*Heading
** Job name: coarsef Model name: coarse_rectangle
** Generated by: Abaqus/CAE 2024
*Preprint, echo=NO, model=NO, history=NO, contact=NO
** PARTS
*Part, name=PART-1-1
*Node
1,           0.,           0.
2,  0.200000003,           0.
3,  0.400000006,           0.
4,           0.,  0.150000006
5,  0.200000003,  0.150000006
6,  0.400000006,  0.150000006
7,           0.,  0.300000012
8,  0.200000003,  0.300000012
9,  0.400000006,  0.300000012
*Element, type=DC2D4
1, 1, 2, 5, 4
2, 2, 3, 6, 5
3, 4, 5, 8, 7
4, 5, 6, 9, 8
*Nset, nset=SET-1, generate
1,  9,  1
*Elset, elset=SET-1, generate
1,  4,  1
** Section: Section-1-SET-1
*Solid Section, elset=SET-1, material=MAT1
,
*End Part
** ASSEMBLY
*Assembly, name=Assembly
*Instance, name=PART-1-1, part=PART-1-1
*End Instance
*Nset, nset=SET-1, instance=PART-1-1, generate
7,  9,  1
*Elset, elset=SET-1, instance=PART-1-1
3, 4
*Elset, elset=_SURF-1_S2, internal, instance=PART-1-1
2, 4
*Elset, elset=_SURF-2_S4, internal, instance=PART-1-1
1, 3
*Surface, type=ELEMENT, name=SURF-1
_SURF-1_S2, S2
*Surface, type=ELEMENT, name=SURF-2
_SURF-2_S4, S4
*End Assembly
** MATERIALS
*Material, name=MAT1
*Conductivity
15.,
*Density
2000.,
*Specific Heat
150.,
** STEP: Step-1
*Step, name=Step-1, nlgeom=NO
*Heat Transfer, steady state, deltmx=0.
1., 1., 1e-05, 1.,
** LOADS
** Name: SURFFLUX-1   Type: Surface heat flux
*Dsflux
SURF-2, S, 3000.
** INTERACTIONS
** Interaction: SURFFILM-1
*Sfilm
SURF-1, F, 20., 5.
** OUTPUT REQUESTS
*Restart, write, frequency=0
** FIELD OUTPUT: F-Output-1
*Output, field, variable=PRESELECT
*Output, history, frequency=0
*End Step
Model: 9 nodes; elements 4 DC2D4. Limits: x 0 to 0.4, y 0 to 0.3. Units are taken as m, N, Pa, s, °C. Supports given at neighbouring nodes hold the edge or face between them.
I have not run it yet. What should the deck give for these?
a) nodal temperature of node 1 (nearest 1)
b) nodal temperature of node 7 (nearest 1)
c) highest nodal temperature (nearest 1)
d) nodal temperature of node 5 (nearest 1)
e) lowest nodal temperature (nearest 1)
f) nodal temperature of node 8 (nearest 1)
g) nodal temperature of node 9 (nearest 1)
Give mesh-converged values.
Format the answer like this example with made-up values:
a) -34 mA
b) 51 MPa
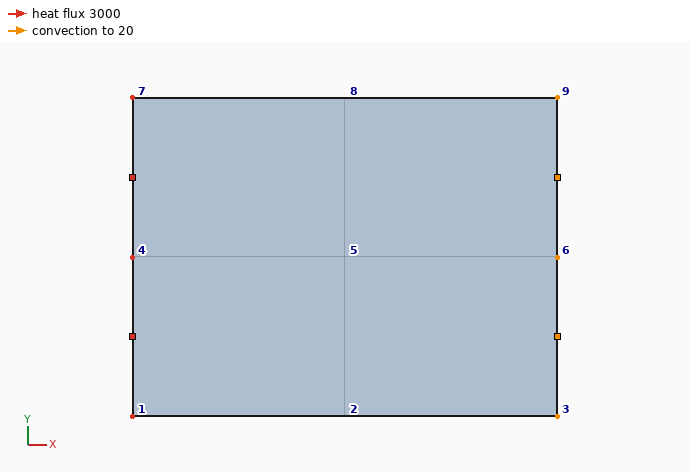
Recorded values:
a) 700 °C
b) 700 °C
c) 700 °C
d) 660 °C
e) 620 °C
f) 660 °C
g) 620 °C
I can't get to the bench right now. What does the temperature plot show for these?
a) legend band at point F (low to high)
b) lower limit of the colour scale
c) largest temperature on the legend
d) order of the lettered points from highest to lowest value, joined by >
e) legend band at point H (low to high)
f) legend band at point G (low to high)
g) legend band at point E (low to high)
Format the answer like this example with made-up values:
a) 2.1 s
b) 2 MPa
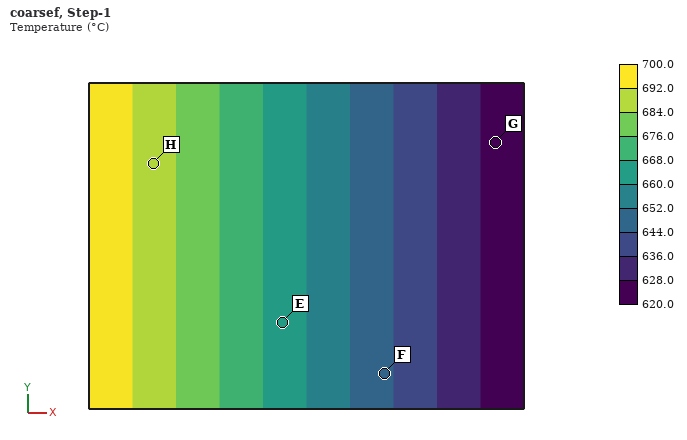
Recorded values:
a) 644.0 to 652.0 °C
b) 620.0 °C
c) 700.0 °C
d) H > E > F > G
e) 684.0 to 692.0 °C
f) 620.0 to 628.0 °C
g) 660.0 to 668.0 °C
